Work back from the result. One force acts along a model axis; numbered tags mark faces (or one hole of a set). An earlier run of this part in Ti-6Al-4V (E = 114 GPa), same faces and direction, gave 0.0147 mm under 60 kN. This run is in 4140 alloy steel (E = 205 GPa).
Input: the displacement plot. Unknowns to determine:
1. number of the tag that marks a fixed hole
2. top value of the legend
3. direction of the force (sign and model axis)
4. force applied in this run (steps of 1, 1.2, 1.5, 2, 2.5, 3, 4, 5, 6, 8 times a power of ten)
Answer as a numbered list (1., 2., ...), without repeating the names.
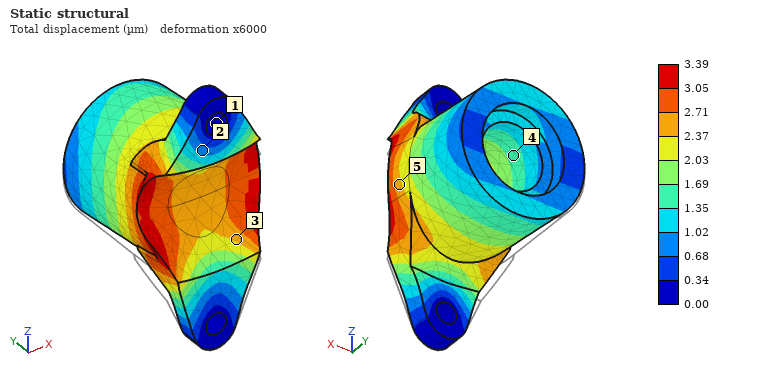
1. 1
2. 3.39 µm
3. +Z
4. 25 kN
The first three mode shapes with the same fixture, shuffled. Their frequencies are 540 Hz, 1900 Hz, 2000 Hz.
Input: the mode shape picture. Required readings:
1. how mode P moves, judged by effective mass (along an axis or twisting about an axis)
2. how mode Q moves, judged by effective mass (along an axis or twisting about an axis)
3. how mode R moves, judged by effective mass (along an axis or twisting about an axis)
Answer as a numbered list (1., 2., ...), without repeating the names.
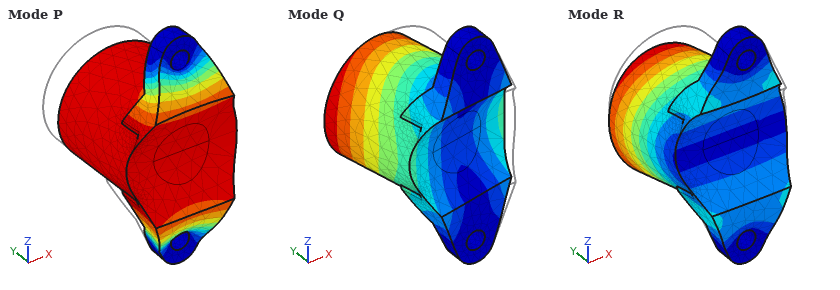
1. along Y
2. along X
3. along Z
